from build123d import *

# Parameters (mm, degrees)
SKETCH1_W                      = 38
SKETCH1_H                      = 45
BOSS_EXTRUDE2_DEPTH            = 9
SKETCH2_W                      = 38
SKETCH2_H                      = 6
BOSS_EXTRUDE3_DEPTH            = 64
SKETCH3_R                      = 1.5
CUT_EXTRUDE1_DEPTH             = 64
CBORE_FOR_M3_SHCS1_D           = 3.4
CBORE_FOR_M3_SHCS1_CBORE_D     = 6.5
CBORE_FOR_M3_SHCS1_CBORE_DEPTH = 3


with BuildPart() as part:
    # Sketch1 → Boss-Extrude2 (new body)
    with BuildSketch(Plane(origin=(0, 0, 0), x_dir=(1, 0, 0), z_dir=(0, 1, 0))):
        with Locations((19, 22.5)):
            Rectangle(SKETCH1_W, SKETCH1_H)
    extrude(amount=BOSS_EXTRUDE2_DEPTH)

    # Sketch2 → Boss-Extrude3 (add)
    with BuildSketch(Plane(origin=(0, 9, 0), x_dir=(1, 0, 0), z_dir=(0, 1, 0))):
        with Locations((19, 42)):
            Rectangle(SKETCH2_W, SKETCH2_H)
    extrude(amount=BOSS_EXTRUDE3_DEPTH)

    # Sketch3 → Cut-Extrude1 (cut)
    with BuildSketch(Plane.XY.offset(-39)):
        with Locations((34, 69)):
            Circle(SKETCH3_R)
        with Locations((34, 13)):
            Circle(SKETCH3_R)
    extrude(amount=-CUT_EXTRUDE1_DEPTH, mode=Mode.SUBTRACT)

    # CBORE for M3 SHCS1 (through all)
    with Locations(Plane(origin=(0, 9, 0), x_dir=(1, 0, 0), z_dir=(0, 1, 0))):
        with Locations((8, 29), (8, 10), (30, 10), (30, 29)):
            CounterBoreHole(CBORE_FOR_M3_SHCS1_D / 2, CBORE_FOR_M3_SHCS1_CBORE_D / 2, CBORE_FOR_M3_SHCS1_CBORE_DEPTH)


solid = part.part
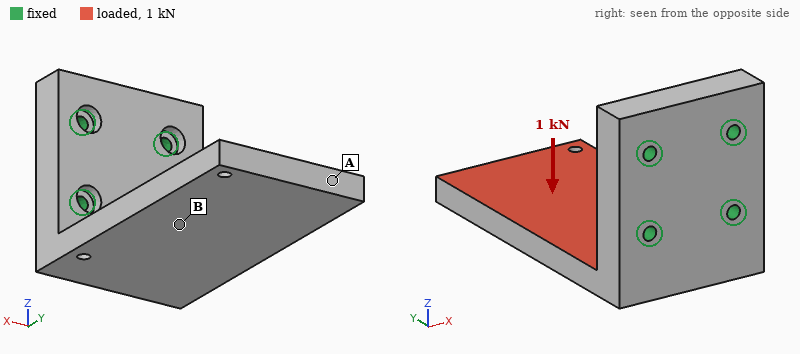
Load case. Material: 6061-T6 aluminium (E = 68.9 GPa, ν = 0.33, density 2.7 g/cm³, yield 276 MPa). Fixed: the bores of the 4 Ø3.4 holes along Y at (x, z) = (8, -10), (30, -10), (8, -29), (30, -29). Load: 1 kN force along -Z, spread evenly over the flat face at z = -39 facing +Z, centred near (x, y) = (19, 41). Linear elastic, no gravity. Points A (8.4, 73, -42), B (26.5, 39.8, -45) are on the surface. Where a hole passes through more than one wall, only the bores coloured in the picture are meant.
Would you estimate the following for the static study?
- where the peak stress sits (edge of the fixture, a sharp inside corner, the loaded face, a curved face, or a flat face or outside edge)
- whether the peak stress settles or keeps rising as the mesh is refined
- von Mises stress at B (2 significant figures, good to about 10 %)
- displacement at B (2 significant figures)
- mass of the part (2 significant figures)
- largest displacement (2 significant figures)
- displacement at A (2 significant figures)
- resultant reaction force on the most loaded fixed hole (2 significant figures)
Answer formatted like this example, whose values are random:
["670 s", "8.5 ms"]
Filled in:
["edge of the fixture", "keeps rising", "37 MPa", "0.43 mm", "79 g", "1.1 mm", "1.1 mm", "890 N"]
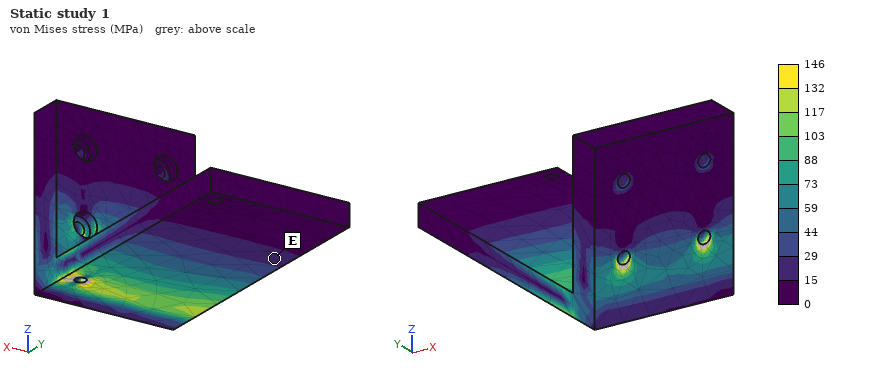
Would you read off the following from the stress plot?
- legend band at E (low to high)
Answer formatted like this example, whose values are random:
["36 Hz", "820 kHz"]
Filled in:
["15 to 29 MPa"]
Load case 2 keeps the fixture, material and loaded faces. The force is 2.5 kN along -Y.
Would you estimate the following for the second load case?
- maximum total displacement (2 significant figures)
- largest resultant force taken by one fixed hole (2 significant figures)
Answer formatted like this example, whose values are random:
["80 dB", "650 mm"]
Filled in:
["0.13 mm", "1.6 kN"]
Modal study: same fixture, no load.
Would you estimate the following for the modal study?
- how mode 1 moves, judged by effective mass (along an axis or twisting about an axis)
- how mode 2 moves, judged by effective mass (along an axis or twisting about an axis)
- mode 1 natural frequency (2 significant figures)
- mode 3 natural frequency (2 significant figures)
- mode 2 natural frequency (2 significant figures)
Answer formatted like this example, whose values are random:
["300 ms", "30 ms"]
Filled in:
["along Z", "along X", "970 Hz", "4000 Hz", "2700 Hz"]
